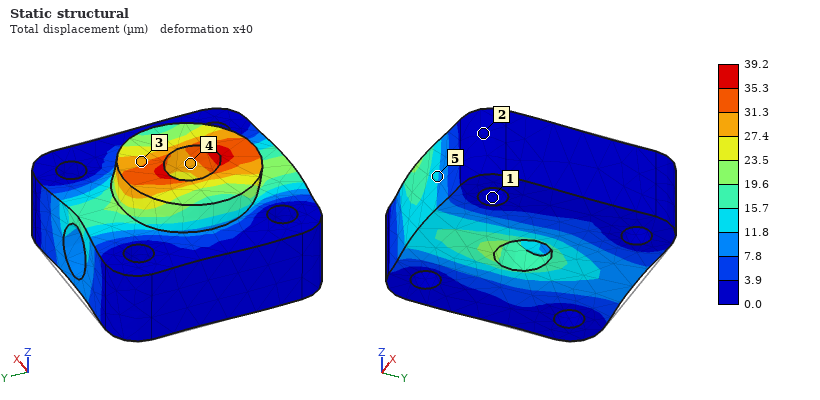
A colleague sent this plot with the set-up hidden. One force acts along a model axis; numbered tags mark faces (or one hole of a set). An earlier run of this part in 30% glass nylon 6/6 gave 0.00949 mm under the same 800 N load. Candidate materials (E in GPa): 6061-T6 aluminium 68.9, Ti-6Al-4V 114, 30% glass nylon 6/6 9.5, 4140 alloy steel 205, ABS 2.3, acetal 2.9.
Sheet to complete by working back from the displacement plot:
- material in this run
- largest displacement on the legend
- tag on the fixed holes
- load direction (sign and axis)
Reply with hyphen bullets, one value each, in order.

- ABS
- 39.2 µm
- 1
- -Y
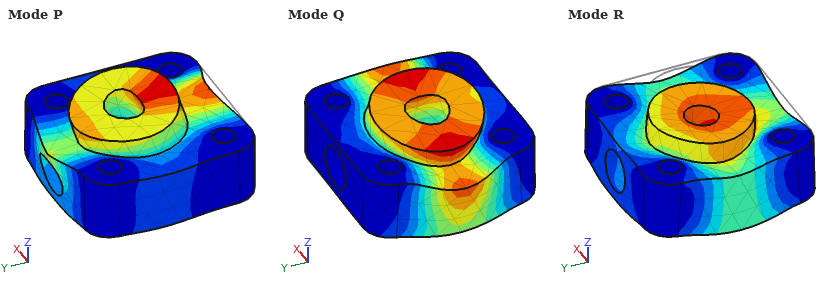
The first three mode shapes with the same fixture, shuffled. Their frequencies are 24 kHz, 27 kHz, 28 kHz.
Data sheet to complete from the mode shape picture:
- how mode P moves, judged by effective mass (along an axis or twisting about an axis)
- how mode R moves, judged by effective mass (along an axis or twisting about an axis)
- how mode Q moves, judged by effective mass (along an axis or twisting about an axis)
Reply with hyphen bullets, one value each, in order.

- along Y
- along Z
- along X
